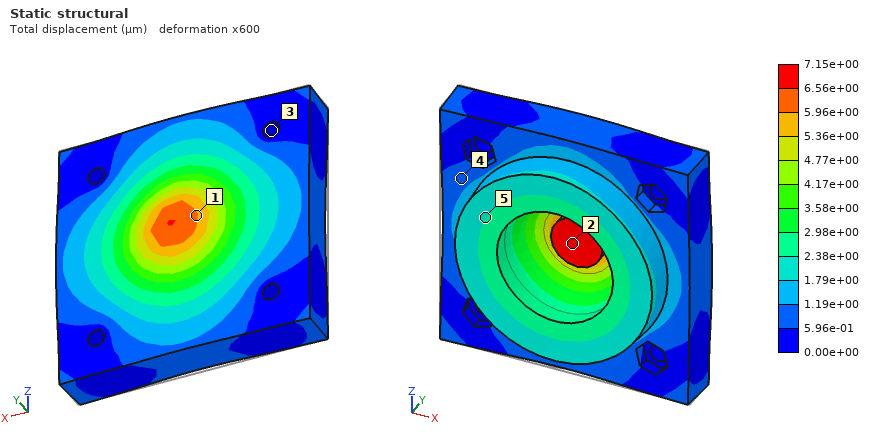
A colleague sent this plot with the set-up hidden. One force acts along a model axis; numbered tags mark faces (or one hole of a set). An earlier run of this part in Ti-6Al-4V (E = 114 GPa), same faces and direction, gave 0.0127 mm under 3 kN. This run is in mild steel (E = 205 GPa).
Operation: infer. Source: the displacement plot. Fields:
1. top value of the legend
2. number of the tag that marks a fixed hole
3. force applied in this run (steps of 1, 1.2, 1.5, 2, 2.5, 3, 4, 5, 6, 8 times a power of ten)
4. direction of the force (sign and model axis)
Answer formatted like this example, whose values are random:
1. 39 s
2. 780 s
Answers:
1. 7.15e+00 µm
2. 3
3. 3 kN
4. +Y
